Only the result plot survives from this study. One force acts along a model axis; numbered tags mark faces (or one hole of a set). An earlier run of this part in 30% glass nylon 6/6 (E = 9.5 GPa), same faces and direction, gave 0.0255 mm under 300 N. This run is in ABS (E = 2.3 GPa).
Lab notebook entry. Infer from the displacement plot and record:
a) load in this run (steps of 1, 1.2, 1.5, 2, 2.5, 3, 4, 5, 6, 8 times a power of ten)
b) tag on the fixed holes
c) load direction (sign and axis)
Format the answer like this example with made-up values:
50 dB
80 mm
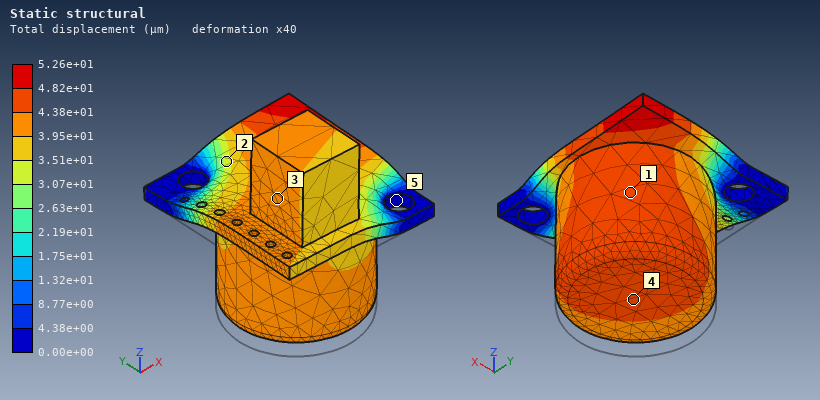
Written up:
150 N
5
+Z
